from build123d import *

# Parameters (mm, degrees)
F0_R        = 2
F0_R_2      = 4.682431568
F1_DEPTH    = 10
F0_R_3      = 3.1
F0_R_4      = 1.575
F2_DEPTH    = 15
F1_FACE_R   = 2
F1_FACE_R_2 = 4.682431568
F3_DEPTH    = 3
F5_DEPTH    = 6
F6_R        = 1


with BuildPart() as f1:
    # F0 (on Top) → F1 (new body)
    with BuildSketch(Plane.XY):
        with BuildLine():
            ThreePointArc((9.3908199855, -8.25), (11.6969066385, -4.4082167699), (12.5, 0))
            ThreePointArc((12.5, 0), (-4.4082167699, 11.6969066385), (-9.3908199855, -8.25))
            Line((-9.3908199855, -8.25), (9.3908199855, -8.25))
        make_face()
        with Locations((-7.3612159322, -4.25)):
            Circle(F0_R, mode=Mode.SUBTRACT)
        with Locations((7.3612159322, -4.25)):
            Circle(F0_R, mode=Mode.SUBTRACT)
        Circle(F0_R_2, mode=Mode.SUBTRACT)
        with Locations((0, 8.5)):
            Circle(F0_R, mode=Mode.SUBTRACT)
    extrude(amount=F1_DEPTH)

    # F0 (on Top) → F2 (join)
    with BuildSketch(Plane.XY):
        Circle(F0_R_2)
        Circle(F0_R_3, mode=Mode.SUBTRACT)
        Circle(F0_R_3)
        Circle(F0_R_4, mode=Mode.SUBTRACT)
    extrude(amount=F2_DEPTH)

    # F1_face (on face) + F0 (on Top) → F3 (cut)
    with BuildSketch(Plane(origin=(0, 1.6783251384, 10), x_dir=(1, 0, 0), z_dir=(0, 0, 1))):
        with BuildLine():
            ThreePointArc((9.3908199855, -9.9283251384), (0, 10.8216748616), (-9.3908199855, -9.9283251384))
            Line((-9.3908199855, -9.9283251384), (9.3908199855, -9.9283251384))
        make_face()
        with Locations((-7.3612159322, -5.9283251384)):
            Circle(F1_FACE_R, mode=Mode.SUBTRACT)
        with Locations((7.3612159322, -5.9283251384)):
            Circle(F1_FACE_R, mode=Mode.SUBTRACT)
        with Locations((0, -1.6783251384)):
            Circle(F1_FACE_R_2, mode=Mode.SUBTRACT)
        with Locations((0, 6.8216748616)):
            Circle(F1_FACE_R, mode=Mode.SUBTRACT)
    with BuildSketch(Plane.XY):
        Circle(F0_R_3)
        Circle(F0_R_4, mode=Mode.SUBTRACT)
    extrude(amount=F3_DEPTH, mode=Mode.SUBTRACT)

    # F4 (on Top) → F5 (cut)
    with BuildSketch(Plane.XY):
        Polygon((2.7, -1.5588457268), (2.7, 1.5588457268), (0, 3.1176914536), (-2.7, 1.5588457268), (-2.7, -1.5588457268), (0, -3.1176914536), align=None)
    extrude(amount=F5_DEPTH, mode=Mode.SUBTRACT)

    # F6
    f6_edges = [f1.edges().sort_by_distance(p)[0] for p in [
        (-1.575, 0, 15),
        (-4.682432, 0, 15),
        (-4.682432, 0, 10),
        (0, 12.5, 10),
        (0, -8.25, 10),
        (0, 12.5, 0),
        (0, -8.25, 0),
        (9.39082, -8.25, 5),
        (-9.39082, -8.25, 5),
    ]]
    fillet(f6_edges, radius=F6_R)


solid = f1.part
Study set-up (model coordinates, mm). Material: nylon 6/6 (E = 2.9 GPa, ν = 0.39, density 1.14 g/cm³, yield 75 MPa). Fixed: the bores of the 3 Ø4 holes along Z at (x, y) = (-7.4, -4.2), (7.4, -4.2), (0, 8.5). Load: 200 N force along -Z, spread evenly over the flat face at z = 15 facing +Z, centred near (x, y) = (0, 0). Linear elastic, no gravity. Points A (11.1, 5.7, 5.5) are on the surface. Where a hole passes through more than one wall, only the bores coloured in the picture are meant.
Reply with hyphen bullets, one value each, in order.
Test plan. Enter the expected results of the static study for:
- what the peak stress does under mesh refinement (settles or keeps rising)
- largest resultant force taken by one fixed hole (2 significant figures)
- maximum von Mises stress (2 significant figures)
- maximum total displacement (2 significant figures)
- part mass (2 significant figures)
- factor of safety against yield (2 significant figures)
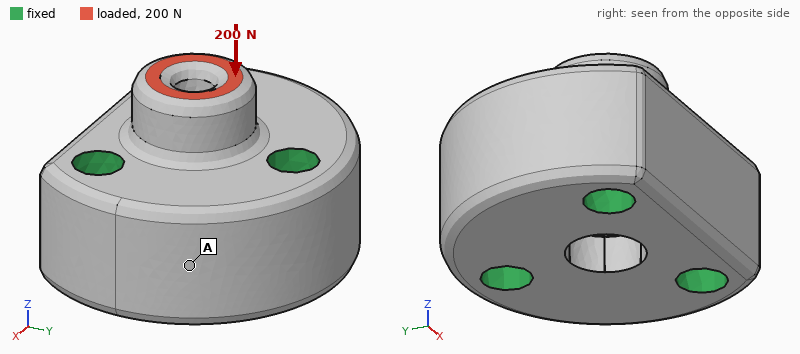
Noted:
- settles
- 74 N
- 6.8 MPa
- 11 µm
- 4.6 g
- 11
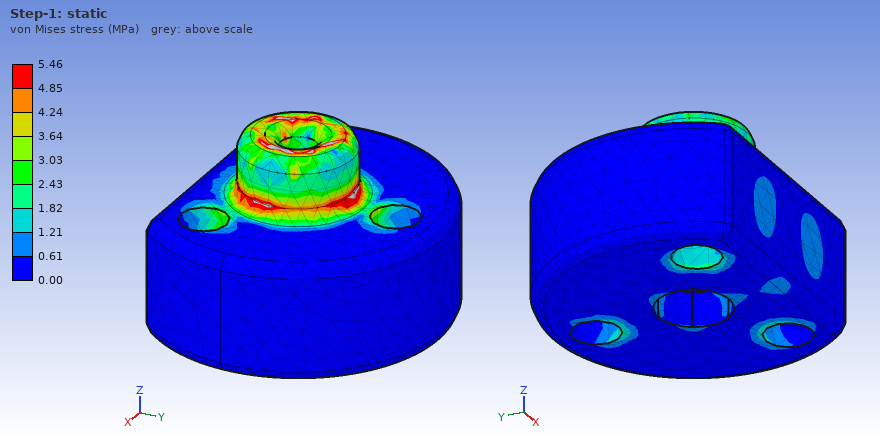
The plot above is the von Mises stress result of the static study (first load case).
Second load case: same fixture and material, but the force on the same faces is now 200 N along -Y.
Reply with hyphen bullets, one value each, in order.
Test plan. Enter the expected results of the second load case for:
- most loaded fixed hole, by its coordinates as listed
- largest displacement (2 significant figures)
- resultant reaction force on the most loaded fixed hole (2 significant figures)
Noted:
- (0, 8.5)
- 49 µm
- 140 N
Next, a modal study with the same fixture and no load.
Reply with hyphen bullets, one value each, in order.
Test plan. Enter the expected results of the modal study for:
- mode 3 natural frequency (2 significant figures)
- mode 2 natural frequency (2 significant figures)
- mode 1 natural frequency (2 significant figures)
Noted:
- 27 kHz
- 24 kHz
- 23 kHz
